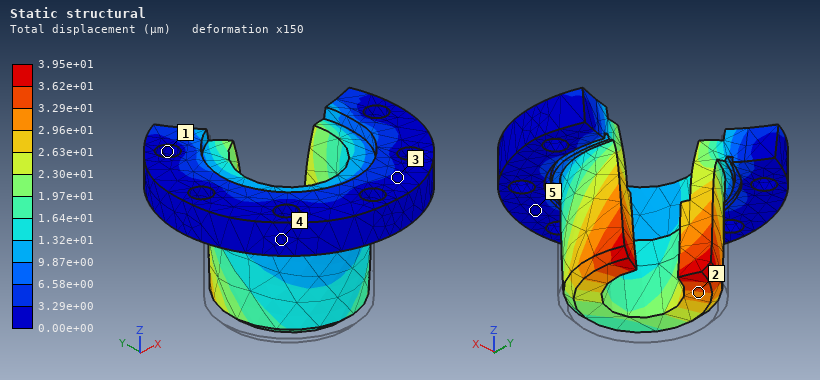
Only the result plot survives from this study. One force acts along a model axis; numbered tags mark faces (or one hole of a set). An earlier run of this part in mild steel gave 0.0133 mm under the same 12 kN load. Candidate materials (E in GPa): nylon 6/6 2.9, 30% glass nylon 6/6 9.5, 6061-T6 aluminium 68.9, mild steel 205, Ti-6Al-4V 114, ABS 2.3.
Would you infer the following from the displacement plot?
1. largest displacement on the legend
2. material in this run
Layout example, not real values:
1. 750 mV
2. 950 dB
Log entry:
1. 3.95e+01 µm
2. 6061-T6 aluminium
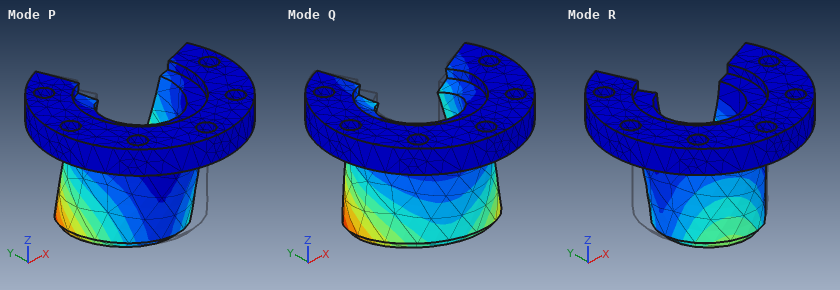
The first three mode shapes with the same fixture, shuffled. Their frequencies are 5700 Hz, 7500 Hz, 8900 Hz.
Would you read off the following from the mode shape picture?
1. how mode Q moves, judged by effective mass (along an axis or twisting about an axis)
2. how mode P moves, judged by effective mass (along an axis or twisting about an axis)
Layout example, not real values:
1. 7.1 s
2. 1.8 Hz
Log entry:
1. along Y
2. along X
